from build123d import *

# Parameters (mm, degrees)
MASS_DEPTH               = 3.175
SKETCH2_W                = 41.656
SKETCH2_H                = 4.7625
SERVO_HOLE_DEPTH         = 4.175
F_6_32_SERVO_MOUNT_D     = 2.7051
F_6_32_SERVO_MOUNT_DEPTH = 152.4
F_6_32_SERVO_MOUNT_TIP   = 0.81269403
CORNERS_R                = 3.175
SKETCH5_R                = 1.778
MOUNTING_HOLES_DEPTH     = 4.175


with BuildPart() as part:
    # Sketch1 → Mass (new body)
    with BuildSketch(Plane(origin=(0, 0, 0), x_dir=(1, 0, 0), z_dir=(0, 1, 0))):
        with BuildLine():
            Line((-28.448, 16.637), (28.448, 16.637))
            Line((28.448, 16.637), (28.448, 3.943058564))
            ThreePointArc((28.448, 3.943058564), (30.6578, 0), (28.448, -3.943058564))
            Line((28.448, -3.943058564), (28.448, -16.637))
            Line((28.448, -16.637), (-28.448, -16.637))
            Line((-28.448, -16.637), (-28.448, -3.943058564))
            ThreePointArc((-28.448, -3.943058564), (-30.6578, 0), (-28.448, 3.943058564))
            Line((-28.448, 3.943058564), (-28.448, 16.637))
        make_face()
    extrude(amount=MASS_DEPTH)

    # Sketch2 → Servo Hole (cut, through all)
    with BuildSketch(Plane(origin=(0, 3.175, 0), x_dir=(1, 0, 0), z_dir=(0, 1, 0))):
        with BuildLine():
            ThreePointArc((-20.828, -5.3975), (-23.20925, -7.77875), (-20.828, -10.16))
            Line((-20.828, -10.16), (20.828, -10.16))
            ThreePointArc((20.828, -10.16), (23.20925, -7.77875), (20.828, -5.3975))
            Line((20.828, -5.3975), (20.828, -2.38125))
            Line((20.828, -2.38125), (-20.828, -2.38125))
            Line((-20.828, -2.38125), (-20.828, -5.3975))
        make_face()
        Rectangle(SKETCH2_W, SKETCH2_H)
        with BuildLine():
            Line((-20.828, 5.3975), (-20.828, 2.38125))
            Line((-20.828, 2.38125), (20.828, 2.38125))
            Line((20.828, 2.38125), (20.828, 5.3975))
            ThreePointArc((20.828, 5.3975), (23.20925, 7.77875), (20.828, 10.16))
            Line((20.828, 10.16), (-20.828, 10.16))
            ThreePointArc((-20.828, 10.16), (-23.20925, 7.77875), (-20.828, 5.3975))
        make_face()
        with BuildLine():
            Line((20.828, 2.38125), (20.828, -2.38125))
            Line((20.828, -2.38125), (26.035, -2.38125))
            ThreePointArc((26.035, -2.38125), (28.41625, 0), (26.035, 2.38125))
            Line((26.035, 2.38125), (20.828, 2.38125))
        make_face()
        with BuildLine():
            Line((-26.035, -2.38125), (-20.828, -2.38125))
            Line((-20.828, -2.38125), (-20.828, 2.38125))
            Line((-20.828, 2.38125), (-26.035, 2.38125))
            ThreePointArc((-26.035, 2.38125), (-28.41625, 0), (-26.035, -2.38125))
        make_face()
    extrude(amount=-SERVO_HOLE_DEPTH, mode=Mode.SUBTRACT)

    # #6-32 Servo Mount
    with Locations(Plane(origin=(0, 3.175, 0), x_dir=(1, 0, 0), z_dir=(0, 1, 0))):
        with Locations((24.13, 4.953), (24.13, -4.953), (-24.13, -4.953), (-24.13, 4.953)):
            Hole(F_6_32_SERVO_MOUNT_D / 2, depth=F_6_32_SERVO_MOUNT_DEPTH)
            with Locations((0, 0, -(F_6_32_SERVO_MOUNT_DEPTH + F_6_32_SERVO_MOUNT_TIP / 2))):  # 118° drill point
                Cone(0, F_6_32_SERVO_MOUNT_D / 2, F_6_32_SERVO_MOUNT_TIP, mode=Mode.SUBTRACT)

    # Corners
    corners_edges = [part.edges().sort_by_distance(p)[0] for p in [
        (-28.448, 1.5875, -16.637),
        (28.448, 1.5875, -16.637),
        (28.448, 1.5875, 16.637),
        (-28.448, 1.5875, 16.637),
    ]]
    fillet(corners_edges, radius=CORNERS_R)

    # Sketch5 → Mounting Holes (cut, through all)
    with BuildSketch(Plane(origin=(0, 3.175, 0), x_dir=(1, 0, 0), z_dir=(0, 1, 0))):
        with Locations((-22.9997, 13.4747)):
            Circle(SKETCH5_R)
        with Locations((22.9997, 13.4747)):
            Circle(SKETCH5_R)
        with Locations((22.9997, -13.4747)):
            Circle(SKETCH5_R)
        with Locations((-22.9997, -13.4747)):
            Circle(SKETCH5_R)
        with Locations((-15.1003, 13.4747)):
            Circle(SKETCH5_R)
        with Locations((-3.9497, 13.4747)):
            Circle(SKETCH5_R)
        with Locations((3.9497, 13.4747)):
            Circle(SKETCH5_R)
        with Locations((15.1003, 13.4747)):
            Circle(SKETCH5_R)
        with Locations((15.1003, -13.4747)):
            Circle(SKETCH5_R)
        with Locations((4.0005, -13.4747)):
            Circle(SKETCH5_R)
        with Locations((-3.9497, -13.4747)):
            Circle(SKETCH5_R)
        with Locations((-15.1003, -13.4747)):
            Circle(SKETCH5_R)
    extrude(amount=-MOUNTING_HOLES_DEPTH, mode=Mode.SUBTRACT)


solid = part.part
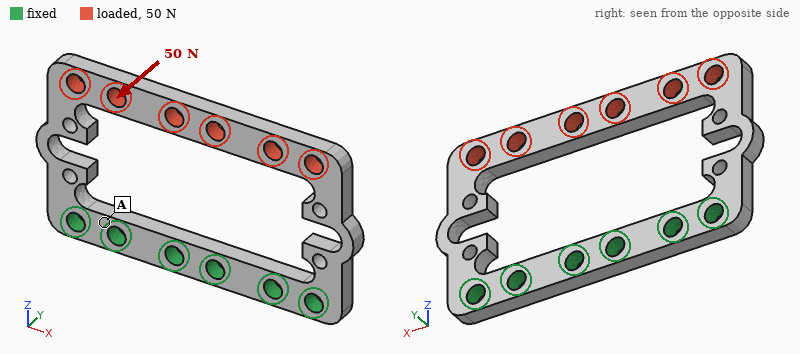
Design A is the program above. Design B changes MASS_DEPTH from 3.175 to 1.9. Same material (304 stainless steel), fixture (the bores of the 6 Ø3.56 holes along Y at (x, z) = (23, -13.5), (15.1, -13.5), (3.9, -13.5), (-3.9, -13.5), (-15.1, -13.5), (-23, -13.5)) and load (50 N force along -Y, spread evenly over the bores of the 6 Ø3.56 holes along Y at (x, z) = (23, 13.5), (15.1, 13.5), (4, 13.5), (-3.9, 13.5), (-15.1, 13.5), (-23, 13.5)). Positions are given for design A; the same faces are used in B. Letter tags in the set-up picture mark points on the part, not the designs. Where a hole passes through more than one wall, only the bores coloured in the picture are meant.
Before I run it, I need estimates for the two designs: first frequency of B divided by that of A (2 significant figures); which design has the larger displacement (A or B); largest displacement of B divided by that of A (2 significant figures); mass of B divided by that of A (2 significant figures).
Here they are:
0.64
B
4.1
0.60
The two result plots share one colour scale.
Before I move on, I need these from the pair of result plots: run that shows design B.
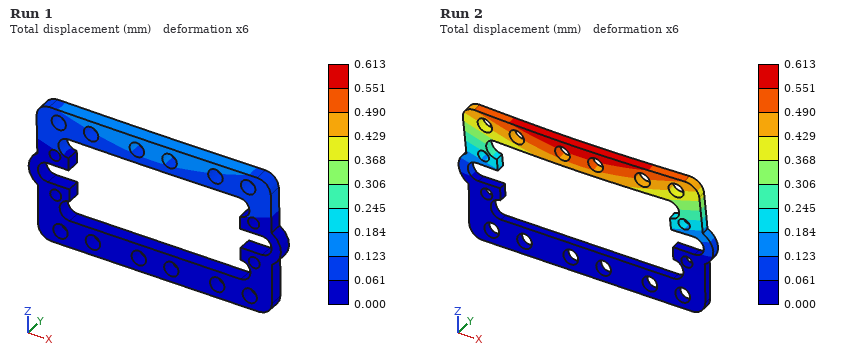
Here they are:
Run 2
